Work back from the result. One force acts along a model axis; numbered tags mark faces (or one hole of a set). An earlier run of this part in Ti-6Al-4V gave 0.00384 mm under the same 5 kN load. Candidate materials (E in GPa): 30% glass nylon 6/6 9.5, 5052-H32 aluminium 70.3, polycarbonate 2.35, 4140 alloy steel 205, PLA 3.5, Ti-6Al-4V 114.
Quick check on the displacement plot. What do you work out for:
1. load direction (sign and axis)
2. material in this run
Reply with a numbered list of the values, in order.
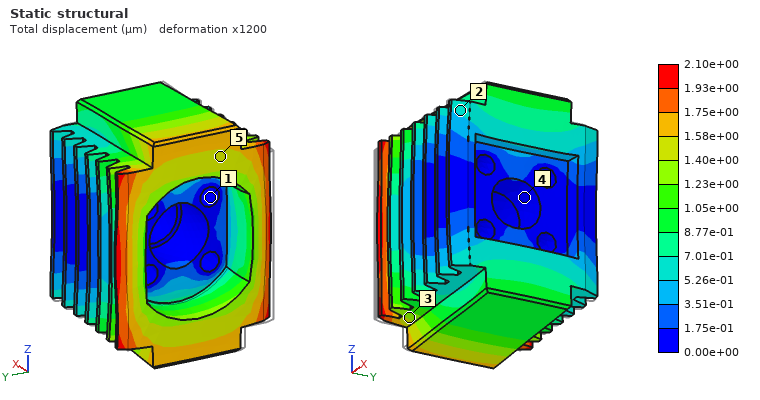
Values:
1. +X
2. 4140 alloy steel
